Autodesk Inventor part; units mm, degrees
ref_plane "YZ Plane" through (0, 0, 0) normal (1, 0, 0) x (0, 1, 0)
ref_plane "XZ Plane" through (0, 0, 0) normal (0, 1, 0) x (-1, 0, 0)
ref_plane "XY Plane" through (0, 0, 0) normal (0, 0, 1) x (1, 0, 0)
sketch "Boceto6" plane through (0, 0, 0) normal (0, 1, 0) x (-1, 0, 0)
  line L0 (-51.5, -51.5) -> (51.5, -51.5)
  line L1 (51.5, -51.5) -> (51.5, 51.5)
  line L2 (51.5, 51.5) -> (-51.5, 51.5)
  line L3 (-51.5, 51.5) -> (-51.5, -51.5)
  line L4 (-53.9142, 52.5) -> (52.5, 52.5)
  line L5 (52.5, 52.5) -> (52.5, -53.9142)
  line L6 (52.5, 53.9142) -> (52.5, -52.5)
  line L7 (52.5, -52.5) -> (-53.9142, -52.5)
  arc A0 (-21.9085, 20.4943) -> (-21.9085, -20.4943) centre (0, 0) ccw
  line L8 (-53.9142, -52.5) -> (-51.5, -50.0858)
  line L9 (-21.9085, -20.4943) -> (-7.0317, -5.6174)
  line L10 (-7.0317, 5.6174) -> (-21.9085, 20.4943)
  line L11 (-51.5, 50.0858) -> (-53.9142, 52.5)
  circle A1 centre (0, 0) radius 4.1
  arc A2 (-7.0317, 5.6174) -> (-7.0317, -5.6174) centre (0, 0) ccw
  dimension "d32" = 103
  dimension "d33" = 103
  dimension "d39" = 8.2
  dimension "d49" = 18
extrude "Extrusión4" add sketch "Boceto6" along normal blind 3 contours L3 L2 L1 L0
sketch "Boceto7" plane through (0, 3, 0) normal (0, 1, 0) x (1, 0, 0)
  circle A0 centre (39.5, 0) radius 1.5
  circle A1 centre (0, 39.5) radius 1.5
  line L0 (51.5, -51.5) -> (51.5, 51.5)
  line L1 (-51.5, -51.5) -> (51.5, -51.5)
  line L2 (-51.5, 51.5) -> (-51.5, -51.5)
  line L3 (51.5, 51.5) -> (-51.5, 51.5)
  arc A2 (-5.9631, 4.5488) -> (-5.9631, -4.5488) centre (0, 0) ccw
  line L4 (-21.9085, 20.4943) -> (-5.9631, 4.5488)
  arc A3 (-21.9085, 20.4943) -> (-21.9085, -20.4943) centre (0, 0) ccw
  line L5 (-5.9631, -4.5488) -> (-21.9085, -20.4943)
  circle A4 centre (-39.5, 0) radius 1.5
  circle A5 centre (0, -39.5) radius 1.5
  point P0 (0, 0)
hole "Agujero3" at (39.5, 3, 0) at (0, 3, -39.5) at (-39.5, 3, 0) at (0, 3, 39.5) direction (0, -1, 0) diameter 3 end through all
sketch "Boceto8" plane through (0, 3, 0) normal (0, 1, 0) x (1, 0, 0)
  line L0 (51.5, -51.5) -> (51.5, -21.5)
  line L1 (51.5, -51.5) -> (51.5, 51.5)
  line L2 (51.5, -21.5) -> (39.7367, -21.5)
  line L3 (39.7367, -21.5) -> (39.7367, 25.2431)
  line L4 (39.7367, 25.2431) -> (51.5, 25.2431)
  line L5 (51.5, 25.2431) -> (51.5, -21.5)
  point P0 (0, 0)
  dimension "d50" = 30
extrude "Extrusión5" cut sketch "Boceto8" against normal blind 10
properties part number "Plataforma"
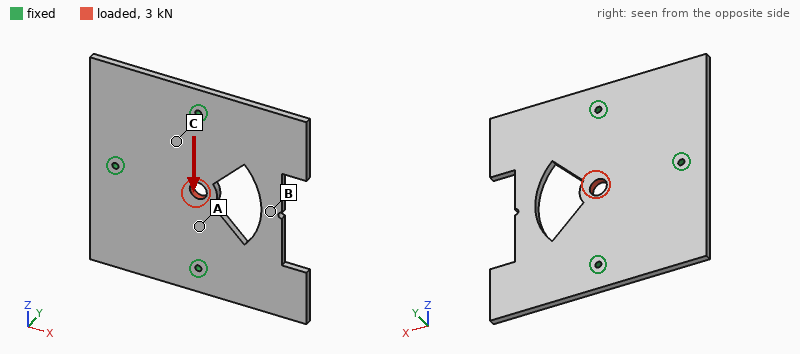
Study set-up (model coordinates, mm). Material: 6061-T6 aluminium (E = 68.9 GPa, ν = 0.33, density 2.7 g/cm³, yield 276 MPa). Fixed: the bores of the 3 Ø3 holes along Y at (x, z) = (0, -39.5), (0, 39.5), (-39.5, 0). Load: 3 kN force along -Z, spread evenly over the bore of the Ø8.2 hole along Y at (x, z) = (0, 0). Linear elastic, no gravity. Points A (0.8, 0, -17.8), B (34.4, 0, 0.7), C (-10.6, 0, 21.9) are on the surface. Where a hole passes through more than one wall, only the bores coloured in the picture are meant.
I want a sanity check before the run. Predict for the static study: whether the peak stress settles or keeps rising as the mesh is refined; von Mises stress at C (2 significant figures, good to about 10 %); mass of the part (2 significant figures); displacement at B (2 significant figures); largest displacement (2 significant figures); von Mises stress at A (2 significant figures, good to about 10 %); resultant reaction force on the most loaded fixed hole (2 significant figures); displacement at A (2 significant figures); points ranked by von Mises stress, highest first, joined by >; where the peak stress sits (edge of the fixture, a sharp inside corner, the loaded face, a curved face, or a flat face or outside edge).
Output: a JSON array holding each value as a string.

["keeps rising", "12 MPa", "76 g", "6.5 µm", "14 µm", "23 MPa", "1.2 kN", "7.6 µm", "A > C > B", "edge of the fixture"]
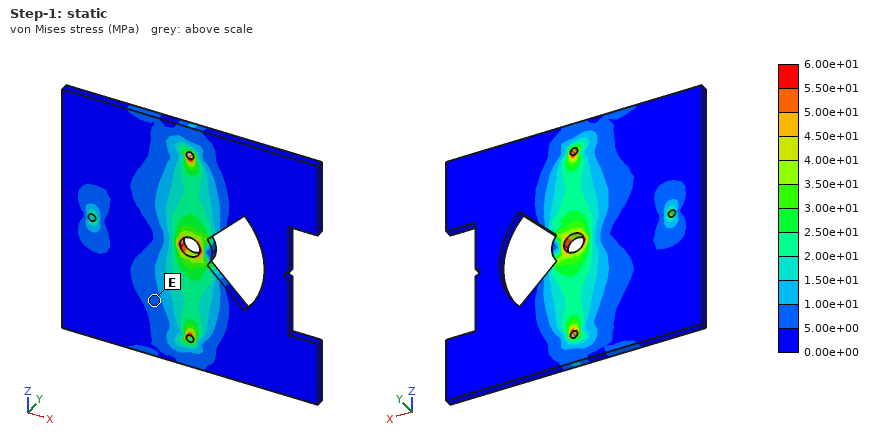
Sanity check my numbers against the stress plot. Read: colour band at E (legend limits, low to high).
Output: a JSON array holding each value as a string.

["5.00e+00 to 1.00e+01 MPa"]
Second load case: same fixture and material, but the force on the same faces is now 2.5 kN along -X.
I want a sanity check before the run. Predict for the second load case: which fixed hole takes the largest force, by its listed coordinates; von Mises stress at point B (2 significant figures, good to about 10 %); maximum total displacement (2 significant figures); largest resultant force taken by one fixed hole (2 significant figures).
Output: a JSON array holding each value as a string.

["(-39.5, 0)", "7.9 MPa", "21 µm", "1.2 kN"]
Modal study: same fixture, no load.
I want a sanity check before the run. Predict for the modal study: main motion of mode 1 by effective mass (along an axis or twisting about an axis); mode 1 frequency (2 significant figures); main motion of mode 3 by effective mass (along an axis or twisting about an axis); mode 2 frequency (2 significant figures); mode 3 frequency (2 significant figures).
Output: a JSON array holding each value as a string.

["along Y", "870 Hz", "twisting about X", "1200 Hz", "1700 Hz"]
